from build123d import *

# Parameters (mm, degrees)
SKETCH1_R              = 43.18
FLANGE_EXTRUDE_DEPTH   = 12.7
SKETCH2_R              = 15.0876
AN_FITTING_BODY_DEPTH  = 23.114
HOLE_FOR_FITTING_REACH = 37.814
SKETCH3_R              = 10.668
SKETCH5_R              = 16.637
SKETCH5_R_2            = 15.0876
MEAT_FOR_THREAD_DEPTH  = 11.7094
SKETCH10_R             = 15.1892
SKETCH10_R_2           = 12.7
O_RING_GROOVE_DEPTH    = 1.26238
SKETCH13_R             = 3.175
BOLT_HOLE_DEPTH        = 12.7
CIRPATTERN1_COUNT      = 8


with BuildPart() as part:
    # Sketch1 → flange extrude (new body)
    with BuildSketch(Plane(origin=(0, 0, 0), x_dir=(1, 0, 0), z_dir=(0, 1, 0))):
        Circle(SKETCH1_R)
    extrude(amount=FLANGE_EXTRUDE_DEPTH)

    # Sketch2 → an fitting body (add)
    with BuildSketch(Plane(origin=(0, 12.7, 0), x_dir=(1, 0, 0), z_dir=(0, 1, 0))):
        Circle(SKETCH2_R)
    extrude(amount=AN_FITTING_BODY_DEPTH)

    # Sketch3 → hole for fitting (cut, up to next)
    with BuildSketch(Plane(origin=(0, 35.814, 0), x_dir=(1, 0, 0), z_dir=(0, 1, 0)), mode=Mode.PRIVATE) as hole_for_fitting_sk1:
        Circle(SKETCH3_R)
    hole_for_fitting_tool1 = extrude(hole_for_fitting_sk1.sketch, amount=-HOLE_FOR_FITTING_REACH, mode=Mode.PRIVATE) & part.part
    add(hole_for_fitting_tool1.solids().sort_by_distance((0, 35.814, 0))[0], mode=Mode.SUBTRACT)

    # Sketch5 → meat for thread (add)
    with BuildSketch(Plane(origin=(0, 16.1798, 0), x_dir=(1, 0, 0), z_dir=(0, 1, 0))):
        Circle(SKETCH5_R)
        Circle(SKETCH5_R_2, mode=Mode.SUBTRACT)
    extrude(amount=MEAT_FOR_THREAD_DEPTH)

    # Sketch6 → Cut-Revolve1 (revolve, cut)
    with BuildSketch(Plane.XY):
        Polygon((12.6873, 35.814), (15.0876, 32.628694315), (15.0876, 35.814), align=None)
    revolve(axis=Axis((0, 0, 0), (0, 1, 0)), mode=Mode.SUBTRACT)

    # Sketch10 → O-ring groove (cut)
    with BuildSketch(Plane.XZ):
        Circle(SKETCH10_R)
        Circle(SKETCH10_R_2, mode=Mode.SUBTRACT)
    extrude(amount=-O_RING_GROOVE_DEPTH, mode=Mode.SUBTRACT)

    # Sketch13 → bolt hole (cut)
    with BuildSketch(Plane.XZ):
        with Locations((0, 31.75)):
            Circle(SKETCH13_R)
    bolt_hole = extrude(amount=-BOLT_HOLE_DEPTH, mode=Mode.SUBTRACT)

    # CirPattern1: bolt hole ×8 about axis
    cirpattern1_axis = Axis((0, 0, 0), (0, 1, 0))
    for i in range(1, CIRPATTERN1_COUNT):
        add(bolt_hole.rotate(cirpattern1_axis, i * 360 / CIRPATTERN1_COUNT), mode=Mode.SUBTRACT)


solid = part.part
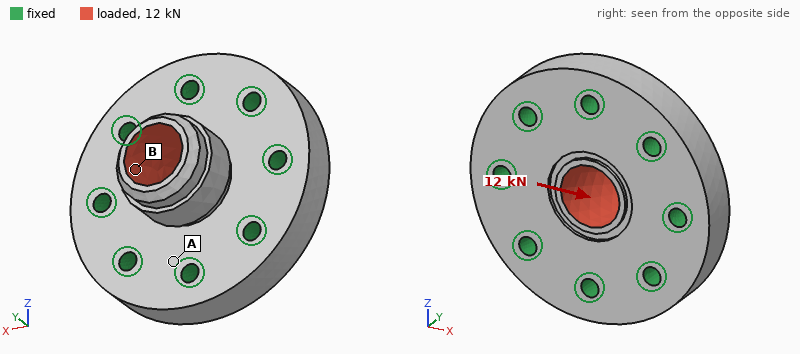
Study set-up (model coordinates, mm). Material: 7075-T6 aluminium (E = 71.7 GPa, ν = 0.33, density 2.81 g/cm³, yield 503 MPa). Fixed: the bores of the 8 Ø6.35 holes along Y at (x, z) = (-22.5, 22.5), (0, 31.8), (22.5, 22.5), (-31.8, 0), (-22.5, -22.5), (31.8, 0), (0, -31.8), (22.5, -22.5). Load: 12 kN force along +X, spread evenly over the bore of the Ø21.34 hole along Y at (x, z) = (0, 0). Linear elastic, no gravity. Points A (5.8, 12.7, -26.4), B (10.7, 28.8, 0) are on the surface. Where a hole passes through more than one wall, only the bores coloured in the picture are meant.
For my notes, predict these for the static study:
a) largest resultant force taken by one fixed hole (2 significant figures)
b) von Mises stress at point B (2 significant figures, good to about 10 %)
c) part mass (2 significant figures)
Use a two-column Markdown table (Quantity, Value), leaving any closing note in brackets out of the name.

| Quantity | Value |
|---|---|
| largest resultant force taken by one fixed hole | 2.9 kN |
| von Mises stress at point B | 19 MPa |
| part mass | 210 g |
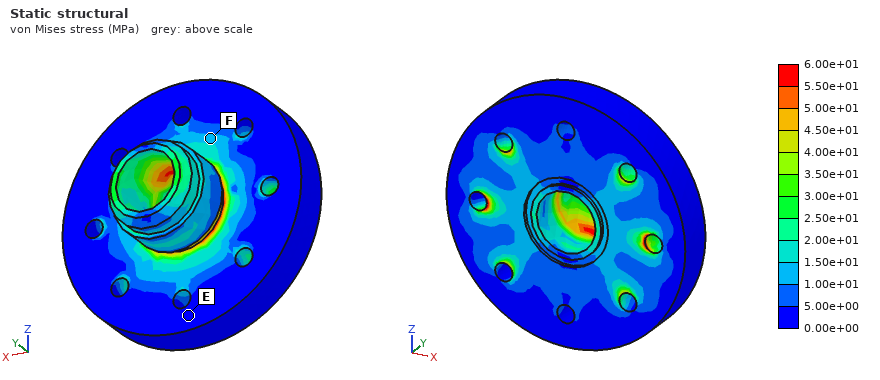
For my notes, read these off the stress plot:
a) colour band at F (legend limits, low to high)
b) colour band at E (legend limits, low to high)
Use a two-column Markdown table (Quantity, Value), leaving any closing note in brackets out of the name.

| Quantity | Value |
|---|---|
| colour band at F | 1.00e+01 to 1.50e+01 MPa |
| colour band at E | 0.00e+00 to 5.00e+00 MPa |
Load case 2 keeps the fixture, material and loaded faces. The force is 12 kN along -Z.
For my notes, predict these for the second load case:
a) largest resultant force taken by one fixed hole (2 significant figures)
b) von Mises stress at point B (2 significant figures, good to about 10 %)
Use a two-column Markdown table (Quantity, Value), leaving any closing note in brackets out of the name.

| Quantity | Value |
|---|---|
| largest resultant force taken by one fixed hole | 2.9 kN |
| von Mises stress at point B | 33 MPa |
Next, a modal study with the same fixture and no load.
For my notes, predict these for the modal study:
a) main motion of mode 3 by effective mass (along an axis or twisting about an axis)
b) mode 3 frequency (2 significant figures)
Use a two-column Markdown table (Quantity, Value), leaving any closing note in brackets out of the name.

| Quantity | Value |
|---|---|
| main motion of mode 3 by effective mass | along Y |
| mode 3 frequency | 20 kHz |
